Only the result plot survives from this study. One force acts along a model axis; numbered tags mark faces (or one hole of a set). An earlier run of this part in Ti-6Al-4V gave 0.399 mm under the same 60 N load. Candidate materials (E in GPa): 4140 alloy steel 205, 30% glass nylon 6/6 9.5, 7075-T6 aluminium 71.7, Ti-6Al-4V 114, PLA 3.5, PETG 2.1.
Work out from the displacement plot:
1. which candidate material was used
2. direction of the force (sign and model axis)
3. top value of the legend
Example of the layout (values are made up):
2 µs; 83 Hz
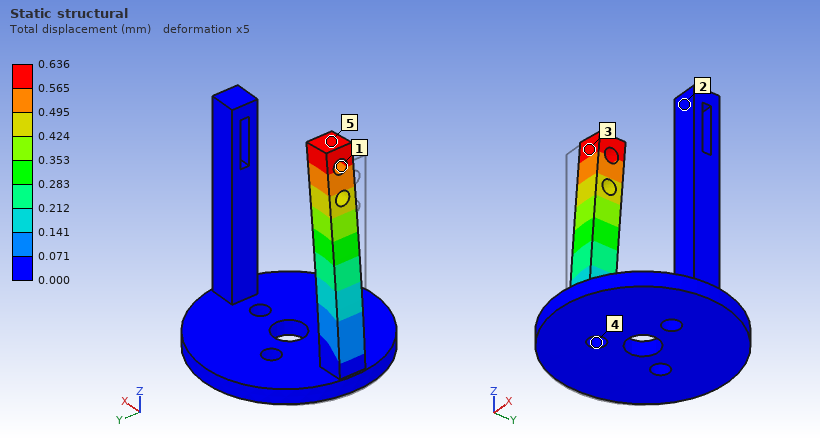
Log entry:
7075-T6 aluminium; +X; 0.636 mm
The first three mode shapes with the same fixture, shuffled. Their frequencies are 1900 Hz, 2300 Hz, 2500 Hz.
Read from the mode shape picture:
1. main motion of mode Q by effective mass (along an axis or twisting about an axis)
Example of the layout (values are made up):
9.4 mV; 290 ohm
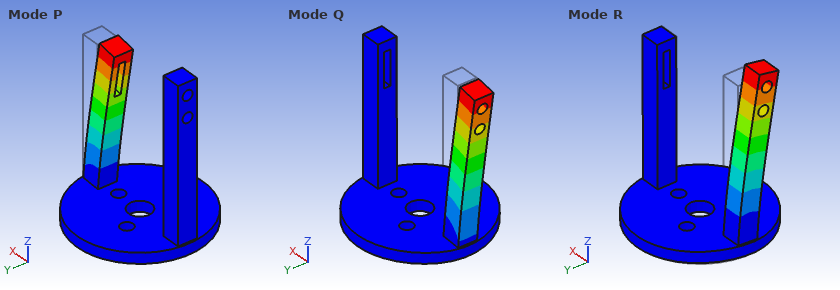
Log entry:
along X
